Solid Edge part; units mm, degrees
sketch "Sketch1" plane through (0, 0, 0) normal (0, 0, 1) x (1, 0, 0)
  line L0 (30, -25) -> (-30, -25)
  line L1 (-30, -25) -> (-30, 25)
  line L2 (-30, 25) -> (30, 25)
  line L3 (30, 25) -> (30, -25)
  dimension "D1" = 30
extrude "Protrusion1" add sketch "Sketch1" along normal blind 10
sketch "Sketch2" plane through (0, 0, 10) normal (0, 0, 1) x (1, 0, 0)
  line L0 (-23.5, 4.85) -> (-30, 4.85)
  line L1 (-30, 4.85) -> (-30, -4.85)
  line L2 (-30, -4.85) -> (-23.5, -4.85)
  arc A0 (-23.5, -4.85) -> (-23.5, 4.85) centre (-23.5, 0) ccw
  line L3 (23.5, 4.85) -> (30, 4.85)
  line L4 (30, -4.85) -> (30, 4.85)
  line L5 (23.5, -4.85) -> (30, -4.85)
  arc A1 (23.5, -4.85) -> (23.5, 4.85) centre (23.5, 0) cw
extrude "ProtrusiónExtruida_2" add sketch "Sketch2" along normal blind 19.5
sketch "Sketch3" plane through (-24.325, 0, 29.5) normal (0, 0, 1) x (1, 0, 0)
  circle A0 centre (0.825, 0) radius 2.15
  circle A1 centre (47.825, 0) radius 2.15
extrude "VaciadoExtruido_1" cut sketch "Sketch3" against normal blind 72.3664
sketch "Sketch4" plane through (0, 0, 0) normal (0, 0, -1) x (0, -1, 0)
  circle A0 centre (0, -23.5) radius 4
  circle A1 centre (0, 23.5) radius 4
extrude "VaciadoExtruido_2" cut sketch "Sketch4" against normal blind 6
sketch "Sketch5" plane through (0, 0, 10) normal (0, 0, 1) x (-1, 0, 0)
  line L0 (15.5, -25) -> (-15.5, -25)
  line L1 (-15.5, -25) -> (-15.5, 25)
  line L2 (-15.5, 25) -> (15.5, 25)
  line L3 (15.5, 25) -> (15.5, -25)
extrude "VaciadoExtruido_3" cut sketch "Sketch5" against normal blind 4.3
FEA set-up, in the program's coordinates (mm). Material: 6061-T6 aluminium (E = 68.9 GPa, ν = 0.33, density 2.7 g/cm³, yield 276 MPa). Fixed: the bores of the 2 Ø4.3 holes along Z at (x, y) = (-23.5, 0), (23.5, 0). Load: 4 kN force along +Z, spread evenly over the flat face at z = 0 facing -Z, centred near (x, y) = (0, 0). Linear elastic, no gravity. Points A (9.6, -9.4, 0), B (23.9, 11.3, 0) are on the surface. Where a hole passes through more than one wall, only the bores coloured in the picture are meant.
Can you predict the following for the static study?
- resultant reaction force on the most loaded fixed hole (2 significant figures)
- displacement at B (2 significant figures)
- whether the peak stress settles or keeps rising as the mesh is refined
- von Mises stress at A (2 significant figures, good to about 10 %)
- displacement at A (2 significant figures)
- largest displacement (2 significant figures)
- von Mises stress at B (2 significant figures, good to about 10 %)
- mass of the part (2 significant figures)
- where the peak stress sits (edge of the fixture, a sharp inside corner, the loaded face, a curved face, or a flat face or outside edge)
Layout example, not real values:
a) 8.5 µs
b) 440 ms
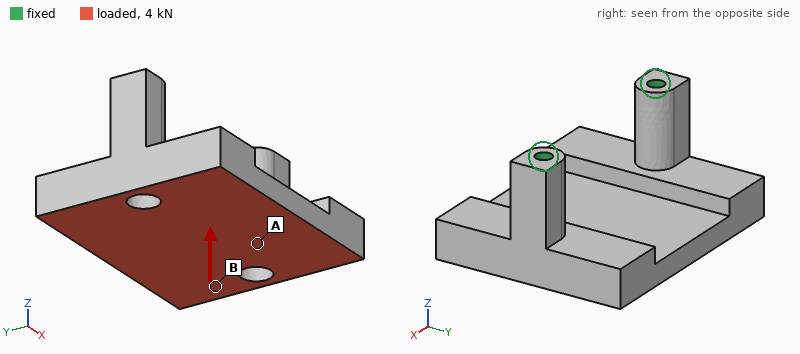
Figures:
a) 2.4 kN
b) 9.0 µm
c) keeps rising
d) 21 MPa
e) 17 µm
f) 37 µm
g) 9.6 MPa
h) 70 g
i) a sharp inside corner
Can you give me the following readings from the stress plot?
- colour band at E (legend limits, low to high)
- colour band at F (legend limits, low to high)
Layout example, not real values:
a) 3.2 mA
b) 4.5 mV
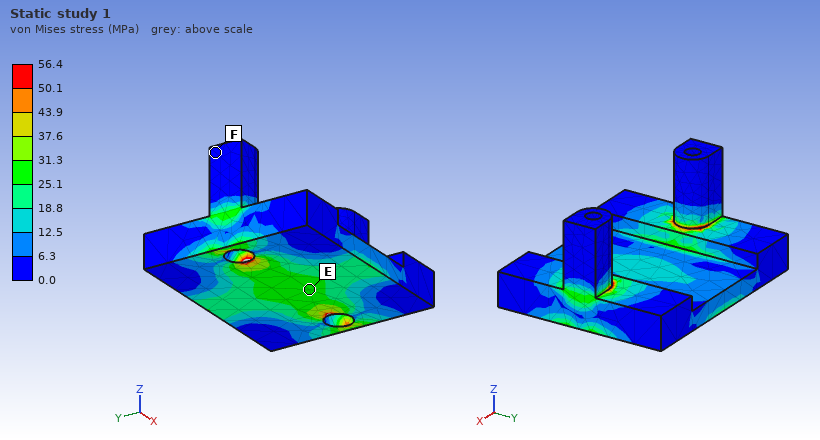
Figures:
a) 25.1 to 31.3 MPa
b) 0.0 to 6.3 MPa
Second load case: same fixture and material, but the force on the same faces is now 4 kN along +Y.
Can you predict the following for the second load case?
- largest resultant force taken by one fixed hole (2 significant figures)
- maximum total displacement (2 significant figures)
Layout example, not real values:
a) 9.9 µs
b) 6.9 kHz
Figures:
a) 2.0 kN
b) 69 µm
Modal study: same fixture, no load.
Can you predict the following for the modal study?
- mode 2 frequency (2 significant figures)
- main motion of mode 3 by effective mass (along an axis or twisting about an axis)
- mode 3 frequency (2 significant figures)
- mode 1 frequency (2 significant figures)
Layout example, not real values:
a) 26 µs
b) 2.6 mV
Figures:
a) 8500 Hz
b) along Z
c) 9600 Hz
d) 5200 Hz
